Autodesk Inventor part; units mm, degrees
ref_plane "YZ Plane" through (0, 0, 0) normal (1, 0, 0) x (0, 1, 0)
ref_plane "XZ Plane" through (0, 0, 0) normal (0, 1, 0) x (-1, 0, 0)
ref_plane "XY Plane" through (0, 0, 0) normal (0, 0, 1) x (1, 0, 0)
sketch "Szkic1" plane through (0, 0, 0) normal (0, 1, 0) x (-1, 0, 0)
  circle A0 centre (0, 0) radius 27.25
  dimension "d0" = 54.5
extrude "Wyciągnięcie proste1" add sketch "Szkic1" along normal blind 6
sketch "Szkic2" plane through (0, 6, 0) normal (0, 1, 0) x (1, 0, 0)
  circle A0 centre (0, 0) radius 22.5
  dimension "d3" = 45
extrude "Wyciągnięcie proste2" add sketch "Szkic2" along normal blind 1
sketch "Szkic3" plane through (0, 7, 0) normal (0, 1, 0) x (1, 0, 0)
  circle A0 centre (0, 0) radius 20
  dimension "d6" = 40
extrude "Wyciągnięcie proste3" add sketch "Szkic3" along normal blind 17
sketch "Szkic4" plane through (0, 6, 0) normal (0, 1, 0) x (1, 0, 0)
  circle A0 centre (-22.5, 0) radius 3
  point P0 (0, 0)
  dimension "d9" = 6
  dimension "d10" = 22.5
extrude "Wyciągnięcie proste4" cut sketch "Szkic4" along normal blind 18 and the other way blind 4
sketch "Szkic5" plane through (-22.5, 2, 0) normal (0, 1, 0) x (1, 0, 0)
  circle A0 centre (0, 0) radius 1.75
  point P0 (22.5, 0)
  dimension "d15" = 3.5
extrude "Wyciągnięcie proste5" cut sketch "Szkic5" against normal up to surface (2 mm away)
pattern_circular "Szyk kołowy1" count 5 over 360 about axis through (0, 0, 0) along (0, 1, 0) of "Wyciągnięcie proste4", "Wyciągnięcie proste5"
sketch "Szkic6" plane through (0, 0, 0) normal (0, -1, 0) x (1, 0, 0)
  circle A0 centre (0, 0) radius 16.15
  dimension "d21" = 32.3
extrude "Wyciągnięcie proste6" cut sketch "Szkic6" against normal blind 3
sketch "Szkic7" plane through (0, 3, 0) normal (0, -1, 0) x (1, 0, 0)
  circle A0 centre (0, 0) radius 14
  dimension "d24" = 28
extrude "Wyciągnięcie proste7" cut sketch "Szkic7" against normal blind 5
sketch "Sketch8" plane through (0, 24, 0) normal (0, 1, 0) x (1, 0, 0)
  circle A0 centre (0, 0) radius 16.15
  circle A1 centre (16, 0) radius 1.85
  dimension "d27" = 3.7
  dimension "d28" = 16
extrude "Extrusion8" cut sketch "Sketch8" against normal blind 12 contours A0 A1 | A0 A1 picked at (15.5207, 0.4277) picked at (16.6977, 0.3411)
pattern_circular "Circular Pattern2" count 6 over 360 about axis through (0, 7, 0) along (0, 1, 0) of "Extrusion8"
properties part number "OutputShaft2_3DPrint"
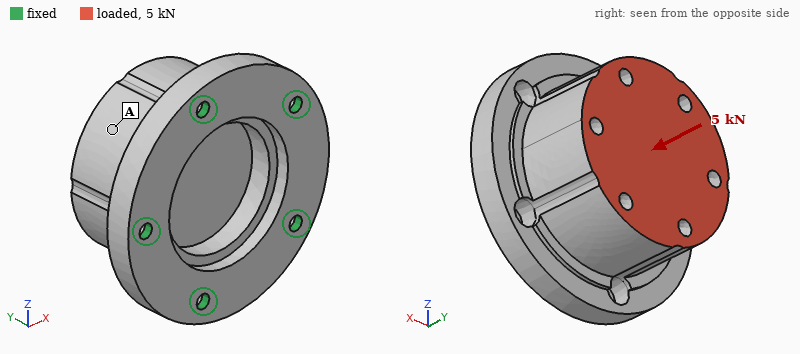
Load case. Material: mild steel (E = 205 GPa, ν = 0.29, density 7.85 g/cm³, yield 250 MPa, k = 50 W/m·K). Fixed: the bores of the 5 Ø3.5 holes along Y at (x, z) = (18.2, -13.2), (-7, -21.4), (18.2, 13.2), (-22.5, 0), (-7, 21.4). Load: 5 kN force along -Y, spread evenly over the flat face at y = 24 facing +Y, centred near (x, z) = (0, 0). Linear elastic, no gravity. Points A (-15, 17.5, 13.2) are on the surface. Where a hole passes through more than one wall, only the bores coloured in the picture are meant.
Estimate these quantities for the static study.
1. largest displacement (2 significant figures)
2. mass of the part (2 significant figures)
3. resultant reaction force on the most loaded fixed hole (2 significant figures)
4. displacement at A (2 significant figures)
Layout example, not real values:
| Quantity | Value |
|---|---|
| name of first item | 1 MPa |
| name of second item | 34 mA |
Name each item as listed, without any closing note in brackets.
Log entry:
| Quantity | Value |
|---|---|
| largest displacement | 2.9 µm |
| mass of the part | 230 g |
| resultant reaction force on the most loaded fixed hole | 1.1 kN |
| displacement at A | 2.6 µm |
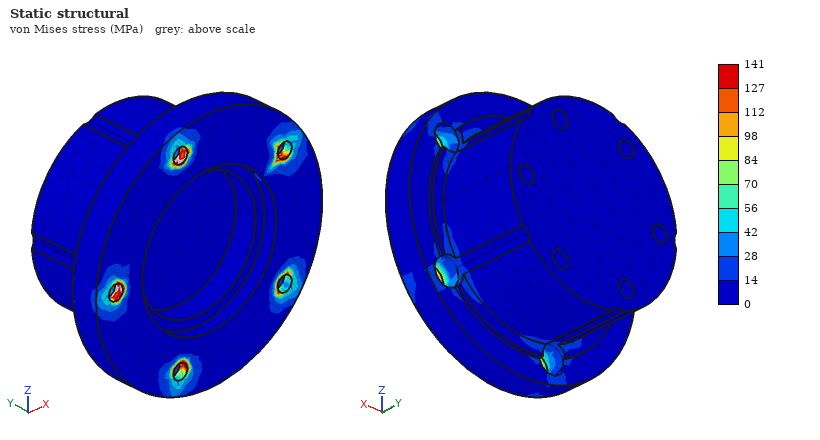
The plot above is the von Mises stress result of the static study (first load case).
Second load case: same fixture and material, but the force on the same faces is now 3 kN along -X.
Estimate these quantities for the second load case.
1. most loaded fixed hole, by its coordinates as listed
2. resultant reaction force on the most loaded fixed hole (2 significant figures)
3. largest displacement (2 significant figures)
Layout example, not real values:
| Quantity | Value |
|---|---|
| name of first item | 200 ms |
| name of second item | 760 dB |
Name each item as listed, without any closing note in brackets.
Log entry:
| Quantity | Value |
|---|---|
| most loaded fixed hole, by its coordinates as listed | (-22.5, 0) |
| resultant reaction force on the most loaded fixed hole | 1.5 kN |
| largest displacement | 5.3 µm |
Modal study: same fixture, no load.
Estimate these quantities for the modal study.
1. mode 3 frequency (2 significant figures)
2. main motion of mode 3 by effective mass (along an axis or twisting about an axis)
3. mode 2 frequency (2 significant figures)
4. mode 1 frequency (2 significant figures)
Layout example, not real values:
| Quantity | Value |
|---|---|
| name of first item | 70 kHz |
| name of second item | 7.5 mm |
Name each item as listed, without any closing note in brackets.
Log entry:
| Quantity | Value |
|---|---|
| mode 3 frequency | 15 kHz |
| main motion of mode 3 by effective mass | along Y |
| mode 2 frequency | 13 kHz |
| mode 1 frequency | 13 kHz |
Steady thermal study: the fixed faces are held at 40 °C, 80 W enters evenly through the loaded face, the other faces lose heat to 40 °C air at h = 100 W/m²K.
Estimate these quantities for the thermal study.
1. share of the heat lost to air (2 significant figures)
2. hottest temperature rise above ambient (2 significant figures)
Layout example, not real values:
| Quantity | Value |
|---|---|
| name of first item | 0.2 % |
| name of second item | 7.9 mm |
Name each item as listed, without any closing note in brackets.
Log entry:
| Quantity | Value |
|---|---|
| share of the heat lost to air | 32 % |
| hottest temperature rise above ambient | 57 K |
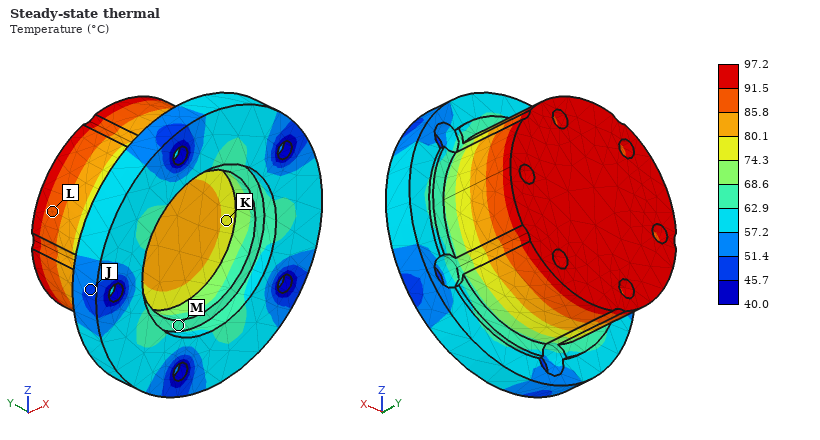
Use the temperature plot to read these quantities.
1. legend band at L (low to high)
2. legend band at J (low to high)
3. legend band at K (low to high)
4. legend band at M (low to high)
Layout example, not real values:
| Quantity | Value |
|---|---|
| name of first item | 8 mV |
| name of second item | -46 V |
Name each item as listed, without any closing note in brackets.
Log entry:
| Quantity | Value |
|---|---|
| legend band at L | 85.8 to 91.5 °C |
| legend band at J | 45.7 to 51.4 °C |
| legend band at K | 74.3 to 80.1 °C |
| legend band at M | 62.9 to 68.6 °C |
